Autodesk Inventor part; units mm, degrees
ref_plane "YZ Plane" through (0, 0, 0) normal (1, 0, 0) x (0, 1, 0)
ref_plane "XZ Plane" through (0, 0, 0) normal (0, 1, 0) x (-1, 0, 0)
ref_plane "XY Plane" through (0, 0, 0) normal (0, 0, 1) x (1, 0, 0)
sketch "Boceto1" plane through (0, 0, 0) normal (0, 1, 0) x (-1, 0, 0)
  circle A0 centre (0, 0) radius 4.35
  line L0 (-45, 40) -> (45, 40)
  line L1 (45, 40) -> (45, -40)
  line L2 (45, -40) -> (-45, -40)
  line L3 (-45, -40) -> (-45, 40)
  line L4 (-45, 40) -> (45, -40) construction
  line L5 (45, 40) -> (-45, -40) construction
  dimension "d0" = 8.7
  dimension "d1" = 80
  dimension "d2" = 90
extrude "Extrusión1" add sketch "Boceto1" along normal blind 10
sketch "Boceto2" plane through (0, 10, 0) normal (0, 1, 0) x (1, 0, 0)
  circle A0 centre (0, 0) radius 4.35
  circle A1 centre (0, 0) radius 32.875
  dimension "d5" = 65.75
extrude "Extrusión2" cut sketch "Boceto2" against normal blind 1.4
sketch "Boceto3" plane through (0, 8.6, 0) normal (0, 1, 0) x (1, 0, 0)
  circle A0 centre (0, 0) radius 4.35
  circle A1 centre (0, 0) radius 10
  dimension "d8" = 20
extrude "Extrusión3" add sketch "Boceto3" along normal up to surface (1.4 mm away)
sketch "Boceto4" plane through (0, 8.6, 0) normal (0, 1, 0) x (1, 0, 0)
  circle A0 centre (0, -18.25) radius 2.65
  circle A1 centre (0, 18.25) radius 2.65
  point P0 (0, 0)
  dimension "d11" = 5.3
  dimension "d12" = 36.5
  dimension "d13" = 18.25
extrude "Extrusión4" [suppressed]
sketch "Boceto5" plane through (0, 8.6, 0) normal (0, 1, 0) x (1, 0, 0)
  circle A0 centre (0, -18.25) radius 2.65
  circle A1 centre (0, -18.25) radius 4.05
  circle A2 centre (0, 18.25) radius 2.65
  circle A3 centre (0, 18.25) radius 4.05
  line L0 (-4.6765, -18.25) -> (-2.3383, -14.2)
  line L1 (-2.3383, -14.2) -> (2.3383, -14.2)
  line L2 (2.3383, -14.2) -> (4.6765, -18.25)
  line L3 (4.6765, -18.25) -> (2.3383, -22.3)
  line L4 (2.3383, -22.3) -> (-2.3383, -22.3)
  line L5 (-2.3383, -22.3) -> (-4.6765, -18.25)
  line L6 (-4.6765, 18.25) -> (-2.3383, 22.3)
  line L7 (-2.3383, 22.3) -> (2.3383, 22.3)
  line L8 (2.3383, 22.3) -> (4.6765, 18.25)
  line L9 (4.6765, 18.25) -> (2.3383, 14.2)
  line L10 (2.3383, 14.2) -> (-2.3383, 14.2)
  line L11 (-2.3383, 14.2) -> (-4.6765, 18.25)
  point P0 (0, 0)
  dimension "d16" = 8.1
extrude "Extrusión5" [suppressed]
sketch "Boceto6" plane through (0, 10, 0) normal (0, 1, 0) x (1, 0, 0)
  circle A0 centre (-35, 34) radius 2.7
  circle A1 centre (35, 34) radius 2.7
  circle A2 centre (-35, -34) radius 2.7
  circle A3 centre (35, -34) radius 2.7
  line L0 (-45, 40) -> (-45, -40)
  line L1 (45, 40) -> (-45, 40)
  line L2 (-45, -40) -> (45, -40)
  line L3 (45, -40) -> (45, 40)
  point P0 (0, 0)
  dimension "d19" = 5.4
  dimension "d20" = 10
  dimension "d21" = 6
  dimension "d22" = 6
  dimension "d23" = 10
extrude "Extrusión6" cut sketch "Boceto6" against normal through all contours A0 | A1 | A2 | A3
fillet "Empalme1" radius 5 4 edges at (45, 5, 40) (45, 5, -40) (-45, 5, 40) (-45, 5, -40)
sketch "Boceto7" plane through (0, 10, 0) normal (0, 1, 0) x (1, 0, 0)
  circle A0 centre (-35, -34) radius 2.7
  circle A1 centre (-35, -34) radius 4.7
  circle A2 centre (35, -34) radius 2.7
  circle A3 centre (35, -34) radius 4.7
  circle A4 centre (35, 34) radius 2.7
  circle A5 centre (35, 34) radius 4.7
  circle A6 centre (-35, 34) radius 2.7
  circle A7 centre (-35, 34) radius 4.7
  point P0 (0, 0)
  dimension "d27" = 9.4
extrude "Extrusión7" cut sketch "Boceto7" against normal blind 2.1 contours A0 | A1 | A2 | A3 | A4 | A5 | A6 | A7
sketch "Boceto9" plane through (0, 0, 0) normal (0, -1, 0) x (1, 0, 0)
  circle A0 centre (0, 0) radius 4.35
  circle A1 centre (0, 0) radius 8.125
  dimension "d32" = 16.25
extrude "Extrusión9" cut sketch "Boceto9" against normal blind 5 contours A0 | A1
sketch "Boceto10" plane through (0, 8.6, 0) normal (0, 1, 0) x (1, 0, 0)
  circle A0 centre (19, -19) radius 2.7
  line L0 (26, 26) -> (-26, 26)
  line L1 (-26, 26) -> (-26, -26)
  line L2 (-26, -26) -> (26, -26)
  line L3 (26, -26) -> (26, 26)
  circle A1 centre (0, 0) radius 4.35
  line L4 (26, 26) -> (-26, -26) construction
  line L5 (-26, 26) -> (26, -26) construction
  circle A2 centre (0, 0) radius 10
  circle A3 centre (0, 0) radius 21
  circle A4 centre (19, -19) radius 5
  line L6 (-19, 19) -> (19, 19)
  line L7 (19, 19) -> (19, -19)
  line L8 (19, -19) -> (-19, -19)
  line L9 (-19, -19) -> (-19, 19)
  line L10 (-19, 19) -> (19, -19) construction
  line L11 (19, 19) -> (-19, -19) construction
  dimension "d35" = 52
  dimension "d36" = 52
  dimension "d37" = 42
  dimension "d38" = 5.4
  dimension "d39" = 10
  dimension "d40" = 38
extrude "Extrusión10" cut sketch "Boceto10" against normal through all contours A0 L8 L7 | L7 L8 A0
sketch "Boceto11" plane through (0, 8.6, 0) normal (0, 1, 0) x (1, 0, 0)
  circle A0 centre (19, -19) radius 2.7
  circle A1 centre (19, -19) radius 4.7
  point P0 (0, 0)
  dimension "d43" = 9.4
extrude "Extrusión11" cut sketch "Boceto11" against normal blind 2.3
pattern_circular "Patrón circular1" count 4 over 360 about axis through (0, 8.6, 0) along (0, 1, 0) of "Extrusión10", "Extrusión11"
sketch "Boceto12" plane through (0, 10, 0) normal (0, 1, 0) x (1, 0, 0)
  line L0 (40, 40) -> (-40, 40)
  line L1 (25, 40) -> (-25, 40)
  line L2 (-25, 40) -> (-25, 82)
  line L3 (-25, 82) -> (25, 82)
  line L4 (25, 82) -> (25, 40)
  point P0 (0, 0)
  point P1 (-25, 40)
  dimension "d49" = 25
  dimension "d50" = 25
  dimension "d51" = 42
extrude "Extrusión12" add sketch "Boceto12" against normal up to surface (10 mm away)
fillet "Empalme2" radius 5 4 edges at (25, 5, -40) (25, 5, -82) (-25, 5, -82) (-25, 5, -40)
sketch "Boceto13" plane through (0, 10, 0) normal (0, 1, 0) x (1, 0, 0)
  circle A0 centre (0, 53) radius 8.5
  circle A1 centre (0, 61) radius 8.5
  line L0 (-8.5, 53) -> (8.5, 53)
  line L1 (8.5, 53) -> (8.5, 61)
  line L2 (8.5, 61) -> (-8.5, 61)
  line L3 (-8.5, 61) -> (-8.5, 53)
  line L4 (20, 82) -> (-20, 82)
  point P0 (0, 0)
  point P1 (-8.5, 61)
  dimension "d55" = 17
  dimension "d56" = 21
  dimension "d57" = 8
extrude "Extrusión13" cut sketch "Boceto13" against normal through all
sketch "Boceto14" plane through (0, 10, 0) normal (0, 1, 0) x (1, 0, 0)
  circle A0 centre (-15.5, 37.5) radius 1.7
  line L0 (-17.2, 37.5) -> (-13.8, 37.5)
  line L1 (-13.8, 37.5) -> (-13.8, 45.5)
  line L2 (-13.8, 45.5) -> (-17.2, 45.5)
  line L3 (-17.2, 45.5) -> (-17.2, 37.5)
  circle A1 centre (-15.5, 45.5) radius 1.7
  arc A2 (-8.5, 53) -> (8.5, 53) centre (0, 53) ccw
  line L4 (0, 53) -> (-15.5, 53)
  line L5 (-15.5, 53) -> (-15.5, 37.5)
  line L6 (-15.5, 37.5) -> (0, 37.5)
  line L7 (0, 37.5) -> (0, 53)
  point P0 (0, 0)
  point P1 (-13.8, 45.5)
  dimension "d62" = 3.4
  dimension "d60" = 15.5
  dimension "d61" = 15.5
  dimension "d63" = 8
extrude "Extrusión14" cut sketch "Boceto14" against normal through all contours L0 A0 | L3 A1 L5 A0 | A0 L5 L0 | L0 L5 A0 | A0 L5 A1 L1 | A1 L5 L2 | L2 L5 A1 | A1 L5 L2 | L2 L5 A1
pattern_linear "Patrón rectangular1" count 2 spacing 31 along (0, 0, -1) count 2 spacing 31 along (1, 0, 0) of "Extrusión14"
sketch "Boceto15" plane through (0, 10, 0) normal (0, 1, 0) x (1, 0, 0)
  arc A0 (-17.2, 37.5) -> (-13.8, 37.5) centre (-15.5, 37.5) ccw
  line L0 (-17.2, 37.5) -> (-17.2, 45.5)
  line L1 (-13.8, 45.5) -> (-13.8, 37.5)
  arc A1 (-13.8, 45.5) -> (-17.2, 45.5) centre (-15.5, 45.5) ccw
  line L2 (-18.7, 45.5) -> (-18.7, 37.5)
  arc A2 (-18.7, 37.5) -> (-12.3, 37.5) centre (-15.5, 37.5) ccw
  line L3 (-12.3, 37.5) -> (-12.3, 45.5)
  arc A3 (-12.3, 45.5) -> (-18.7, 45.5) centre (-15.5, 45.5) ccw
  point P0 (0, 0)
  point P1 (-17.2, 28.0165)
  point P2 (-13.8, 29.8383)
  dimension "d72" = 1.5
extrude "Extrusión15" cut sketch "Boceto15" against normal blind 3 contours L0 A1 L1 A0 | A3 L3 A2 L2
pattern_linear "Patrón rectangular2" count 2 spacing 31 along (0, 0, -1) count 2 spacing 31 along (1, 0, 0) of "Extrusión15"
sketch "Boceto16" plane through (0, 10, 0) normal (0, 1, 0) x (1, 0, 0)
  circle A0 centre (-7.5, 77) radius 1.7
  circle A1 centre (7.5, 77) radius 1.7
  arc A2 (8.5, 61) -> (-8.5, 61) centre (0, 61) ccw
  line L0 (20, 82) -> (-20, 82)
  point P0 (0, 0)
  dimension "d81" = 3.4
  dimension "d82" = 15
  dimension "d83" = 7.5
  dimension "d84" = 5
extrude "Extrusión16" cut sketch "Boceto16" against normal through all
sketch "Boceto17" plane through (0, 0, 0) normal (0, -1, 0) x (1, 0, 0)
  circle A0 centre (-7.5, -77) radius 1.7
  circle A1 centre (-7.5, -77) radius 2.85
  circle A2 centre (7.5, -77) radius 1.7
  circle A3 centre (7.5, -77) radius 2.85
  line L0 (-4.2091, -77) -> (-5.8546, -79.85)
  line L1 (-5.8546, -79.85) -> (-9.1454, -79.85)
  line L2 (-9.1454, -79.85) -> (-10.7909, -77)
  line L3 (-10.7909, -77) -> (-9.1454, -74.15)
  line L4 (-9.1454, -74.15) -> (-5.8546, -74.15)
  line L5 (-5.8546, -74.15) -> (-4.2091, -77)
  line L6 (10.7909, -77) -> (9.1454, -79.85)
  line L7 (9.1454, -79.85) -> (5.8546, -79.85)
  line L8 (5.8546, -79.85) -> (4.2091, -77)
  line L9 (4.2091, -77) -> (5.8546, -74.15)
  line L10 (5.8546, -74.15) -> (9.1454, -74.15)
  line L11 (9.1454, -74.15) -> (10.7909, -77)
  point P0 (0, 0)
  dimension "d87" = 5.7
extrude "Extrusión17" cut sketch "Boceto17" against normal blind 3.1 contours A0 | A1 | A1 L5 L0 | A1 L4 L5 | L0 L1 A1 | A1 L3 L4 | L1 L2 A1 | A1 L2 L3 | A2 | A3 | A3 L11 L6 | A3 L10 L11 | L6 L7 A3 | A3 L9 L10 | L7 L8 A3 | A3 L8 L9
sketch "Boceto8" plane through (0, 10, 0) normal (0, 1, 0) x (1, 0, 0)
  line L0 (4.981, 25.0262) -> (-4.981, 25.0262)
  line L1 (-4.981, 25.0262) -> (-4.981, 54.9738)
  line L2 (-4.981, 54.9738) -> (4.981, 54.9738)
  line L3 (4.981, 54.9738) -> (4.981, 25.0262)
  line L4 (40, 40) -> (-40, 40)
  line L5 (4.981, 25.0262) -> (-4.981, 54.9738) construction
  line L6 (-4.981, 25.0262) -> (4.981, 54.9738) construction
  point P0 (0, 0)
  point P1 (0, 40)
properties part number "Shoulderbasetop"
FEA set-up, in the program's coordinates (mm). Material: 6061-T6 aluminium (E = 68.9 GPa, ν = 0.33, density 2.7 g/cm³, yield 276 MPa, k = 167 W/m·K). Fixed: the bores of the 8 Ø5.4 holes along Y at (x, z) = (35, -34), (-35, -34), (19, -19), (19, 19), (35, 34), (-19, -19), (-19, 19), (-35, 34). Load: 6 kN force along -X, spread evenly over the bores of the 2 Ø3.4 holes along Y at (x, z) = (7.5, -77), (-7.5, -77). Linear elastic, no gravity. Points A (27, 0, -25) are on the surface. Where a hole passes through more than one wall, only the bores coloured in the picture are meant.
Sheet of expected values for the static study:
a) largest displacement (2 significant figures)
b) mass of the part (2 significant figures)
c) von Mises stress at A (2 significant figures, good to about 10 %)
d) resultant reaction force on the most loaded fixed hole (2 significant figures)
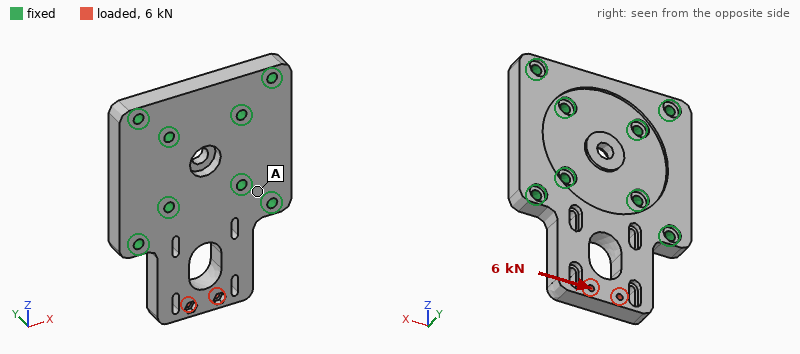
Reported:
0.11 mm
210 g
17 MPa
3.3 kN
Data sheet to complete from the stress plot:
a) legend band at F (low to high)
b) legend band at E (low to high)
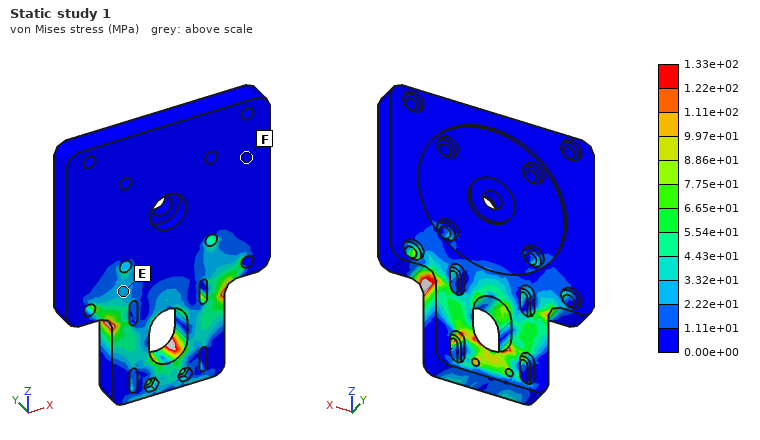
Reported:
0.00e+00 to 1.11e+01 MPa
2.22e+01 to 3.32e+01 MPa
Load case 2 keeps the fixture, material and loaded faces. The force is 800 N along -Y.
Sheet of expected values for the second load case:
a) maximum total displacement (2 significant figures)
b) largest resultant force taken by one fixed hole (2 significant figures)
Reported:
0.22 mm
640 N
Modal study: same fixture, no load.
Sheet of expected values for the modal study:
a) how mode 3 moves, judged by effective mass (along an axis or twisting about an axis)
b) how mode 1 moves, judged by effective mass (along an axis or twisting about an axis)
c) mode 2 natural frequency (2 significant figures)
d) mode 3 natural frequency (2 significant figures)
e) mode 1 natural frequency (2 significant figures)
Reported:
along X
along Y
5800 Hz
9100 Hz
2400 Hz
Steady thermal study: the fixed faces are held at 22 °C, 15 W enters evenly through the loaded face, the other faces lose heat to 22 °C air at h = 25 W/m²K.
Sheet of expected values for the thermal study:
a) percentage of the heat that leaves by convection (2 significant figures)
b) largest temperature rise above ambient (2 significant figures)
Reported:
9.9 %
15 K
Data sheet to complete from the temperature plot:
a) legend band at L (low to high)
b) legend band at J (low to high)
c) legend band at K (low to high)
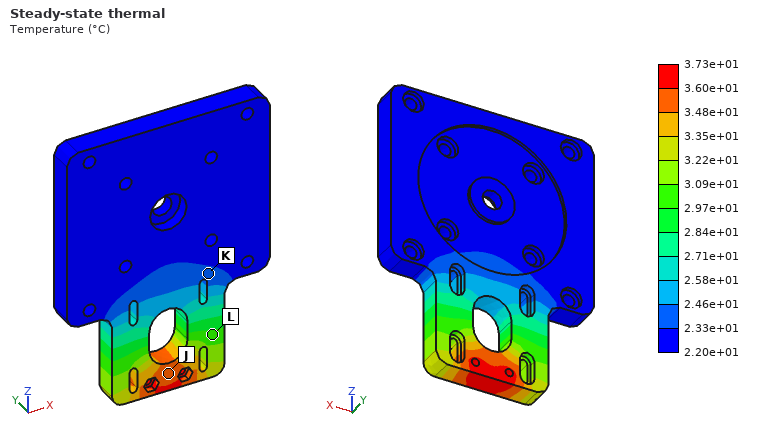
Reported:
2.97e+01 to 3.09e+01 °C
3.48e+01 to 3.60e+01 °C
2.33e+01 to 2.46e+01 °C
